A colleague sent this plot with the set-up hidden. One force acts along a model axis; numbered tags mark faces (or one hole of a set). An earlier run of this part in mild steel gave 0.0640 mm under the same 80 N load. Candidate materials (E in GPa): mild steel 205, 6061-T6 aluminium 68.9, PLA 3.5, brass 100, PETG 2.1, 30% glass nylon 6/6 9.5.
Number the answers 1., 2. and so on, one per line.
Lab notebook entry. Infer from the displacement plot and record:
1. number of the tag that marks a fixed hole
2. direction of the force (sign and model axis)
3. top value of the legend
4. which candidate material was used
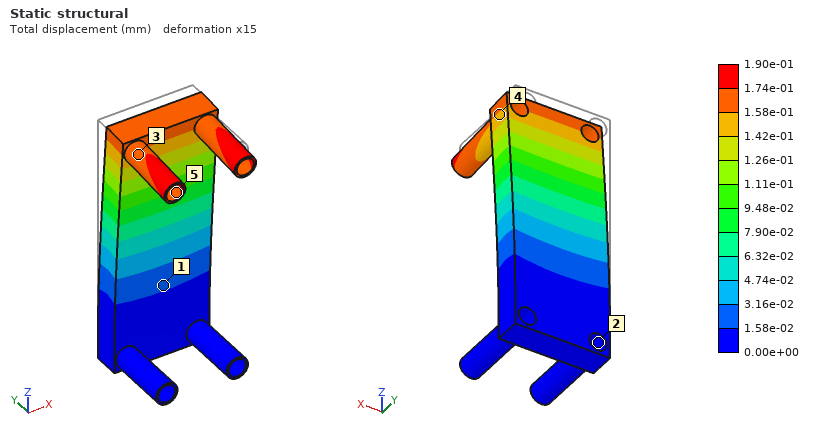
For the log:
1. 2
2. -Y
3. 1.90e-01 mm
4. 6061-T6 aluminium
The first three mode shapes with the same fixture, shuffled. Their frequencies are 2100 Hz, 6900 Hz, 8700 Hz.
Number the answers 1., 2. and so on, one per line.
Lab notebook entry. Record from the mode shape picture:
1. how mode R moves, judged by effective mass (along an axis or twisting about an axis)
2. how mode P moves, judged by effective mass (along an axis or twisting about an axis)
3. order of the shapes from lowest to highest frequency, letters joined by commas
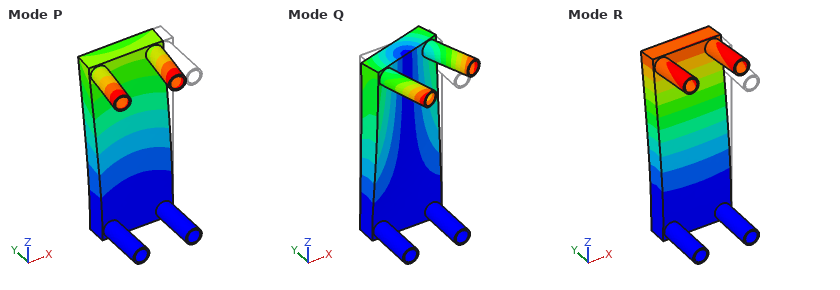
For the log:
1. along Y
2. along X
3. R, P, Q
